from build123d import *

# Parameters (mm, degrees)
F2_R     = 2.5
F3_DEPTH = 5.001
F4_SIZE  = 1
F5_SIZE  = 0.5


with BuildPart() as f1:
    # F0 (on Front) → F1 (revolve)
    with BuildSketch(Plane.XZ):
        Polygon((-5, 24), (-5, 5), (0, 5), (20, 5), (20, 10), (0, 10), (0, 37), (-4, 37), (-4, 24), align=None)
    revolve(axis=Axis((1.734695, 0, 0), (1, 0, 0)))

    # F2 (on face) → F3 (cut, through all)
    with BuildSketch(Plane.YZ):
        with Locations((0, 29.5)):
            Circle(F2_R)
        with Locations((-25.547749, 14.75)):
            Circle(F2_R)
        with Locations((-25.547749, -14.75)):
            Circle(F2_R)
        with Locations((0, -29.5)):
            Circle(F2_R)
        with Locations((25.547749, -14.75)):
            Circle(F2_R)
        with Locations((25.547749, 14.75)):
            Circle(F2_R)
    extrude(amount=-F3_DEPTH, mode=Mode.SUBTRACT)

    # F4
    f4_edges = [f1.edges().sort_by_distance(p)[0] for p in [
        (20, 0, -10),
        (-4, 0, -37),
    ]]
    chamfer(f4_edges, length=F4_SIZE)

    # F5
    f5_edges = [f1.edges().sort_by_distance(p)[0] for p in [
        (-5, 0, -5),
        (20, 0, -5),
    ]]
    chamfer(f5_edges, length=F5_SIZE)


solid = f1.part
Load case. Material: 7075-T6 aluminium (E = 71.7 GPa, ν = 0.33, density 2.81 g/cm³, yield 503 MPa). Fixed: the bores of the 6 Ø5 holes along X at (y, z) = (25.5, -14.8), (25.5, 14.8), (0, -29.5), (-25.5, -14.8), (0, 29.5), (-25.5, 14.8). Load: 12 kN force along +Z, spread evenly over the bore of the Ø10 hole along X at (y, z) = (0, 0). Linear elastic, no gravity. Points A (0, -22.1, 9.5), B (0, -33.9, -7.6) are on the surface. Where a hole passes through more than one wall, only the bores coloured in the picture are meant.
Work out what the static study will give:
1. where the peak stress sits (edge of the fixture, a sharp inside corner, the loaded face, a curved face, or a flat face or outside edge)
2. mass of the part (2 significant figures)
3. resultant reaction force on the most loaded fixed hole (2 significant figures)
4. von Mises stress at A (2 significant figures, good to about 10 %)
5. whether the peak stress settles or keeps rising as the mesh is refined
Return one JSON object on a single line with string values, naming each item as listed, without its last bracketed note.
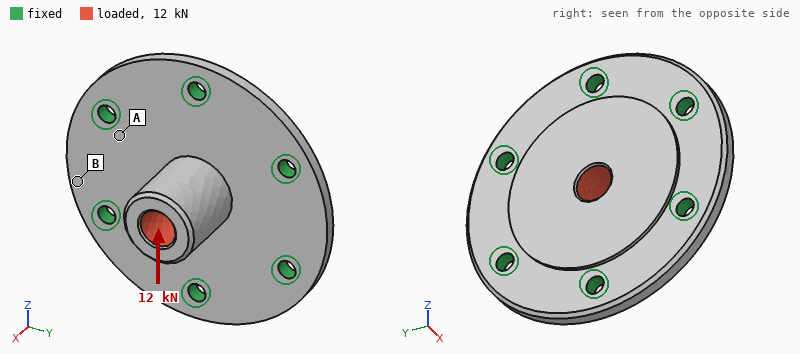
{"where the peak stress sits": "edge of the fixture", "mass of the part": "64 g", "resultant reaction force on the most loaded fixed hole": "3.4 kN", "von Mises stress at A": "68 MPa", "whether the peak stress settles or keeps rising as the mesh is refined": "keeps rising"}
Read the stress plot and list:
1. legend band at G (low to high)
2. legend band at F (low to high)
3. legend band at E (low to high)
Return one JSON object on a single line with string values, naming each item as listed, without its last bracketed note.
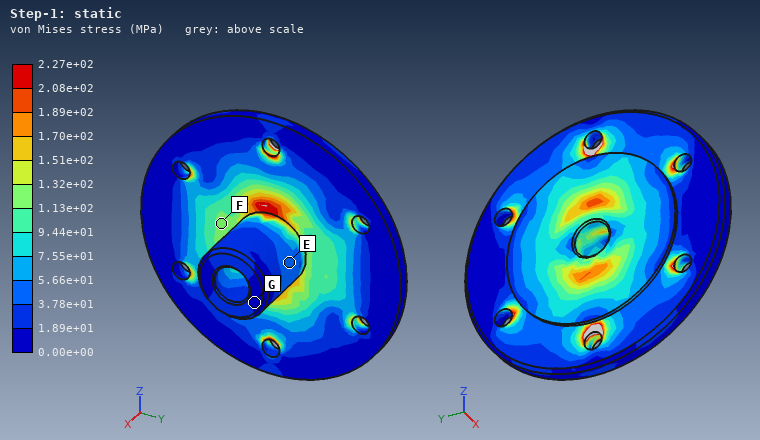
{"legend band at G": "0.00e+00 to 1.89e+01 MPa", "legend band at F": "1.13e+02 to 1.32e+02 MPa", "legend band at E": "3.78e+01 to 5.66e+01 MPa"}
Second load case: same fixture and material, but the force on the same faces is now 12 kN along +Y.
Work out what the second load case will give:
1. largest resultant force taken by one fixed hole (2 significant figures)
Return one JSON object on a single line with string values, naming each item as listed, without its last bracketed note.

{"largest resultant force taken by one fixed hole": "2.9 kN"}
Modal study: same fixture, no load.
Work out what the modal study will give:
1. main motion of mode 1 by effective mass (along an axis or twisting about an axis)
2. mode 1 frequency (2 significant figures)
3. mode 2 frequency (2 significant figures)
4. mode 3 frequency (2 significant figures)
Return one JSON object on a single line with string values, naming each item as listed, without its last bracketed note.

{"main motion of mode 1 by effective mass": "along X", "mode 1 frequency": "8400 Hz", "mode 2 frequency": "9900 Hz", "mode 3 frequency": "9900 Hz"}
